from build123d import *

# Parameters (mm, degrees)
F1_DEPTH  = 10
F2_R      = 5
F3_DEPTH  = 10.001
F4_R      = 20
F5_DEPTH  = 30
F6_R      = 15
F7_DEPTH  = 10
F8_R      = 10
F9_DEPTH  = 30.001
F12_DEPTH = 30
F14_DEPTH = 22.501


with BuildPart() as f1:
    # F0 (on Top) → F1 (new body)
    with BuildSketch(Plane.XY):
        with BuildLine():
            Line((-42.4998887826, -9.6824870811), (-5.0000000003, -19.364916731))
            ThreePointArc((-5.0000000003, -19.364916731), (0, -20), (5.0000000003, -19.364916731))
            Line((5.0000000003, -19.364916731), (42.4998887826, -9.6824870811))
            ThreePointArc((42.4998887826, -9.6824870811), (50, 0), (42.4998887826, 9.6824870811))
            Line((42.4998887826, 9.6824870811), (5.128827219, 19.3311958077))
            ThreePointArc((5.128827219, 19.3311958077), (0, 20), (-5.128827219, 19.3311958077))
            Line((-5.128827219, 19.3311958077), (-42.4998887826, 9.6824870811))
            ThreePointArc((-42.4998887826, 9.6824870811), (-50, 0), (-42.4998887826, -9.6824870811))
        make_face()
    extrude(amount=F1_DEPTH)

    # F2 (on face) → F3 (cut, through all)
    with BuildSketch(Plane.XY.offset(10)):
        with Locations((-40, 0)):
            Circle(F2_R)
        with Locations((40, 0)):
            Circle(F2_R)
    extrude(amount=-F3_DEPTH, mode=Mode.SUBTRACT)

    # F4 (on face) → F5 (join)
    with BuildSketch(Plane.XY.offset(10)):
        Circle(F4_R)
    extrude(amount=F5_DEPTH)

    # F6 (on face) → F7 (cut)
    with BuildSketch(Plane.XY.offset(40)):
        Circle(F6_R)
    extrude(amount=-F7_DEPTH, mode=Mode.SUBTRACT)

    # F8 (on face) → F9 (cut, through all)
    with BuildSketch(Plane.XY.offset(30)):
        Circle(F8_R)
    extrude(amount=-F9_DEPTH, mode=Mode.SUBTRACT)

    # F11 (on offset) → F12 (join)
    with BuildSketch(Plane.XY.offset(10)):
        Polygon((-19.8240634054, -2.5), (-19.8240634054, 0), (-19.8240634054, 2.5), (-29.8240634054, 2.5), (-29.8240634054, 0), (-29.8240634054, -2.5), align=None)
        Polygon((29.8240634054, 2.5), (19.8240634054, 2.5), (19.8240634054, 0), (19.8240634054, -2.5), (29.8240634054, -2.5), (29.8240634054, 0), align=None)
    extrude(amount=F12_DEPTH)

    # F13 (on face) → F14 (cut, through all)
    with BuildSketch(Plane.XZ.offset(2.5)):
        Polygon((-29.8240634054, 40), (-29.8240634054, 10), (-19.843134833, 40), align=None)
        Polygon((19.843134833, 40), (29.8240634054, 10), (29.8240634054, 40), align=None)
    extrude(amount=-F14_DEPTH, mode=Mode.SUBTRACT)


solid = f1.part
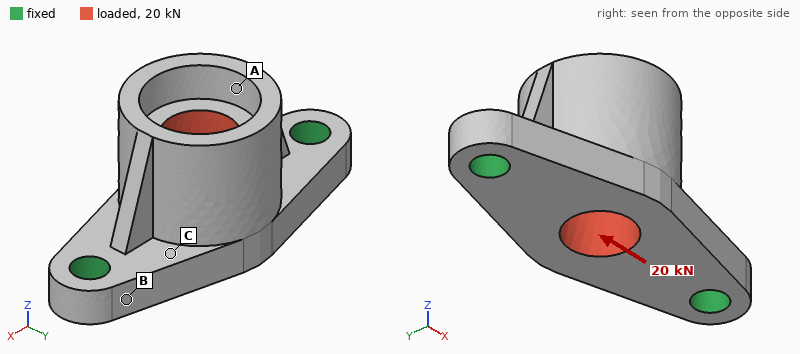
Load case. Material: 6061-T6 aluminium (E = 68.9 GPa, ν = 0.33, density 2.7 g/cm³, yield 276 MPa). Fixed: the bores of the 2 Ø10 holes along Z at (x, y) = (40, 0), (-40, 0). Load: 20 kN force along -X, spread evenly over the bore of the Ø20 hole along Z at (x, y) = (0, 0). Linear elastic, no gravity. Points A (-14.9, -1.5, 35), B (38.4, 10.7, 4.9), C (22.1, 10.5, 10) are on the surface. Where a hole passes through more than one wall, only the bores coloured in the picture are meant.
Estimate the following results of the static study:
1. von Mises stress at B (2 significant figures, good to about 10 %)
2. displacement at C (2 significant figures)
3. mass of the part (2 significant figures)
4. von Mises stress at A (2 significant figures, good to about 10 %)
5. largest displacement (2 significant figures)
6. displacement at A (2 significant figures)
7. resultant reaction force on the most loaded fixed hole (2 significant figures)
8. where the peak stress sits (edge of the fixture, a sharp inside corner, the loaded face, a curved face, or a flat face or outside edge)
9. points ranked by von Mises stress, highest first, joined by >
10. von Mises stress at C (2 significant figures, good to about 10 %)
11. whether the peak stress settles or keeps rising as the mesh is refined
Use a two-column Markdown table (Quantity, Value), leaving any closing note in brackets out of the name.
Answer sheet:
| Quantity | Value |
|---|---|
| von Mises stress at B | 24 MPa |
| displacement at C | 13 µm |
| mass of the part | 130 g |
| von Mises stress at A | 9.9 MPa |
| largest displacement | 38 µm |
| displacement at A | 35 µm |
| resultant reaction force on the most loaded fixed hole | 10 kN |
| where the peak stress sits | edge of the fixture |
| points ranked by von Mises stress, highest first, joined by > | C > B > A |
| von Mises stress at C | 51 MPa |
| whether the peak stress settles or keeps rising as the mesh is refined | keeps rising |
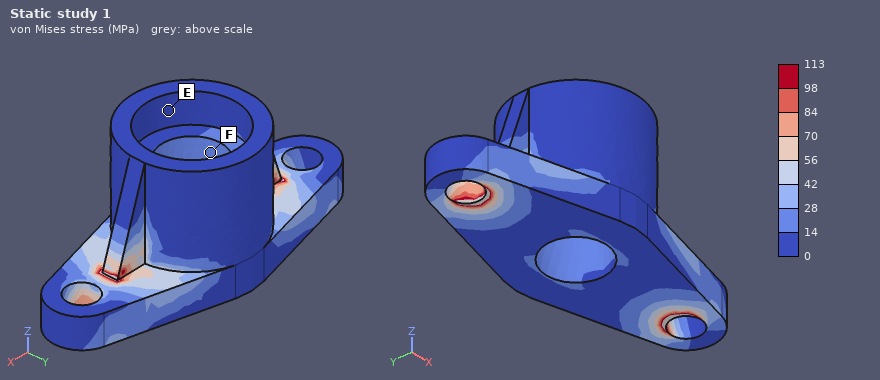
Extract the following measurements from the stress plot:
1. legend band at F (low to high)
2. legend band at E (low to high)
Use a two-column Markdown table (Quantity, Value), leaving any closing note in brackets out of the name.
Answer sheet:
| Quantity | Value |
|---|---|
| legend band at F | 14 to 28 MPa |
| legend band at E | 0 to 14 MPa |
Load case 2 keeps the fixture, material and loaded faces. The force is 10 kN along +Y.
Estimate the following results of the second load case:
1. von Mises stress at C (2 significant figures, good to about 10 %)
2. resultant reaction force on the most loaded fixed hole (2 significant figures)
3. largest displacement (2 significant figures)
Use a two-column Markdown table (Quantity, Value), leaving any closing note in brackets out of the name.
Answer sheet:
| Quantity | Value |
|---|---|
| von Mises stress at C | 71 MPa |
| resultant reaction force on the most loaded fixed hole | 5.0 kN |
| largest displacement | 0.22 mm |
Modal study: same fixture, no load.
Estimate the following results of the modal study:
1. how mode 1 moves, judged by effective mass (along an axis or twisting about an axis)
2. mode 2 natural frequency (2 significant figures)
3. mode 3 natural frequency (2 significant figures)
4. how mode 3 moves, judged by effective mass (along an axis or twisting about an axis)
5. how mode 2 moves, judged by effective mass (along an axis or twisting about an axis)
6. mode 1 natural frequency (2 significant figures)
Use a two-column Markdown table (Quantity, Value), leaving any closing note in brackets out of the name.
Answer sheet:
| Quantity | Value |
|---|---|
| how mode 1 moves, judged by effective mass | along Y |
| mode 2 natural frequency | 7200 Hz |
| mode 3 natural frequency | 11 kHz |
| how mode 3 moves, judged by effective mass | along X |
| how mode 2 moves, judged by effective mass | along Z |
| mode 1 natural frequency | 3400 Hz |
